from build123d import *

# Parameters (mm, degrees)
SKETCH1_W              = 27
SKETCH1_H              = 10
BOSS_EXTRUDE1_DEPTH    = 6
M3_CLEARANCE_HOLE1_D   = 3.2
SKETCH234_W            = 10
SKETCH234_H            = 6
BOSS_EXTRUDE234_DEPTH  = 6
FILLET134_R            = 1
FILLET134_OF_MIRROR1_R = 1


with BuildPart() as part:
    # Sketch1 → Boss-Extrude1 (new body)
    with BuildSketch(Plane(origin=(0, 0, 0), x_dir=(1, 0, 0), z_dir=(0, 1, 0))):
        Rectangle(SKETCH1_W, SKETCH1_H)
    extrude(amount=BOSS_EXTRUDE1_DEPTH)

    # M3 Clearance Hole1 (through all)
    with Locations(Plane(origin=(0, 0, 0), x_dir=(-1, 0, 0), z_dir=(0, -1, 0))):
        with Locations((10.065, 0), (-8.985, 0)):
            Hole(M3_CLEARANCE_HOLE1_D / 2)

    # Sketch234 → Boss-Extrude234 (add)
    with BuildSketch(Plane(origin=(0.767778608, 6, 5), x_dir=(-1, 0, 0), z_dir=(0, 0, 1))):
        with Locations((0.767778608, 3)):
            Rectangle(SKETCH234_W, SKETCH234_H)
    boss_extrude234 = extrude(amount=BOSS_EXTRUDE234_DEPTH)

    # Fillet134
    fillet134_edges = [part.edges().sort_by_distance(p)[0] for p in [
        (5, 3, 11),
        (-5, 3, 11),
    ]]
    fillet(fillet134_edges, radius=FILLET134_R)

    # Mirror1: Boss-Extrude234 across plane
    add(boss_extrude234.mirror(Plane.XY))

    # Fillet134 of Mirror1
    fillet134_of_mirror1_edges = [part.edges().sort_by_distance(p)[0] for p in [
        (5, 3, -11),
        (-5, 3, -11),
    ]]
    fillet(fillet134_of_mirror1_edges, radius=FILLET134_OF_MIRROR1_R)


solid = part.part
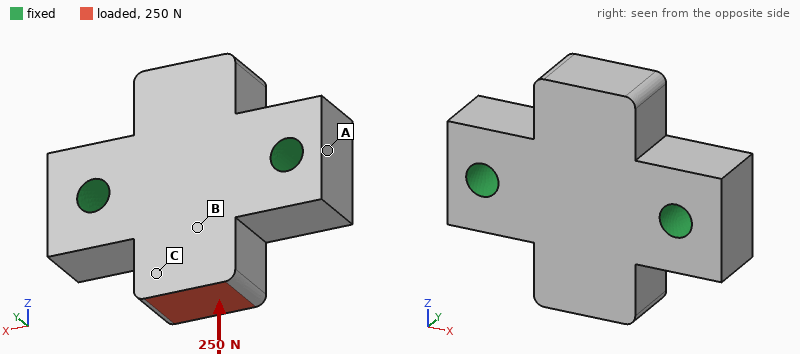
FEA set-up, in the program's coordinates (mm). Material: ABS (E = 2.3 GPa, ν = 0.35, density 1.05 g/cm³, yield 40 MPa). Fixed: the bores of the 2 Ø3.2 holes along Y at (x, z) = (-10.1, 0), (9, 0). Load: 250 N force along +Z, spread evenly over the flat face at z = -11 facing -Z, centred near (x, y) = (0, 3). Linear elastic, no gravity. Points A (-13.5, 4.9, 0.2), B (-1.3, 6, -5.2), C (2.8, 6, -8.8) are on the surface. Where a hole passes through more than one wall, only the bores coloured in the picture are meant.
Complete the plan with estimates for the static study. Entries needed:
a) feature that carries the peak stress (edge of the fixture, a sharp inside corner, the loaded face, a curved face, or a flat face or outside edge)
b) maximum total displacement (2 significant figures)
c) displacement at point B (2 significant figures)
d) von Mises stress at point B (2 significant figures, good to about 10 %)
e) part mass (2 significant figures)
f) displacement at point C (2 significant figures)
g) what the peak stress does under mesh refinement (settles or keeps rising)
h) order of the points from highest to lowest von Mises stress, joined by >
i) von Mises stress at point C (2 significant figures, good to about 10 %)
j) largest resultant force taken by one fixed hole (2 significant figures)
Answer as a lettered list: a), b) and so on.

a) edge of the fixture
b) 34 µm
c) 23 µm
d) 2.8 MPa
e) 2.4 g
f) 27 µm
g) keeps rising
h) C > B > A
i) 5.2 MPa
j) 140 N
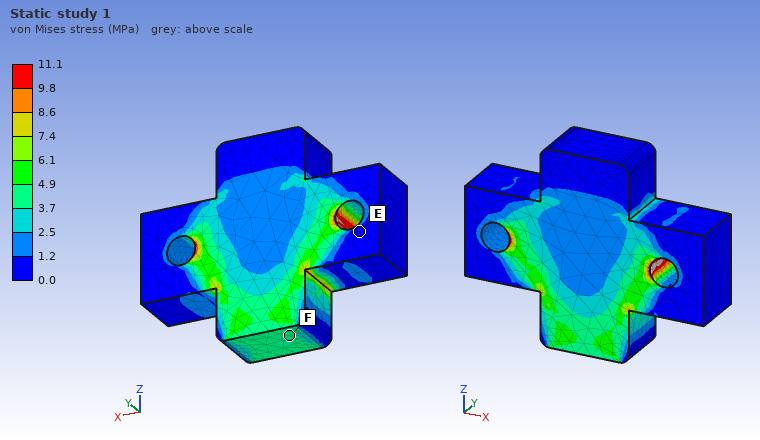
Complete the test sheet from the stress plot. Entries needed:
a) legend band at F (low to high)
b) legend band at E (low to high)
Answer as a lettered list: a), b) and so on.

a) 3.7 to 4.9 MPa
b) 0.0 to 1.2 MPa
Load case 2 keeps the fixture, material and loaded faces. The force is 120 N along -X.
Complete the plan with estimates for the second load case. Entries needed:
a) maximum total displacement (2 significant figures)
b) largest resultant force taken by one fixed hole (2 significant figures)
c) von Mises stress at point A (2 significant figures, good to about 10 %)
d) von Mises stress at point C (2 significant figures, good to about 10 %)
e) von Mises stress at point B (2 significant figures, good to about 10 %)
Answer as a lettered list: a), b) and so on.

a) 49 µm
b) 96 N
c) 0.53 MPa
d) 4.1 MPa
e) 2.6 MPa
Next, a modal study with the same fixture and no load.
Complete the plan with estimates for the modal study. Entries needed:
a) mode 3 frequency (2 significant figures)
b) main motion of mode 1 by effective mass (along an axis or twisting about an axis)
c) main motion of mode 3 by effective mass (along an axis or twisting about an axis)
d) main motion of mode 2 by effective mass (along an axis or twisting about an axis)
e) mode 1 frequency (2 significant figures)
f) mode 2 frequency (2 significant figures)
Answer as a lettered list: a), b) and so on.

a) 15 kHz
b) twisting about X
c) along Z
d) along Y
e) 7400 Hz
f) 9700 Hz
